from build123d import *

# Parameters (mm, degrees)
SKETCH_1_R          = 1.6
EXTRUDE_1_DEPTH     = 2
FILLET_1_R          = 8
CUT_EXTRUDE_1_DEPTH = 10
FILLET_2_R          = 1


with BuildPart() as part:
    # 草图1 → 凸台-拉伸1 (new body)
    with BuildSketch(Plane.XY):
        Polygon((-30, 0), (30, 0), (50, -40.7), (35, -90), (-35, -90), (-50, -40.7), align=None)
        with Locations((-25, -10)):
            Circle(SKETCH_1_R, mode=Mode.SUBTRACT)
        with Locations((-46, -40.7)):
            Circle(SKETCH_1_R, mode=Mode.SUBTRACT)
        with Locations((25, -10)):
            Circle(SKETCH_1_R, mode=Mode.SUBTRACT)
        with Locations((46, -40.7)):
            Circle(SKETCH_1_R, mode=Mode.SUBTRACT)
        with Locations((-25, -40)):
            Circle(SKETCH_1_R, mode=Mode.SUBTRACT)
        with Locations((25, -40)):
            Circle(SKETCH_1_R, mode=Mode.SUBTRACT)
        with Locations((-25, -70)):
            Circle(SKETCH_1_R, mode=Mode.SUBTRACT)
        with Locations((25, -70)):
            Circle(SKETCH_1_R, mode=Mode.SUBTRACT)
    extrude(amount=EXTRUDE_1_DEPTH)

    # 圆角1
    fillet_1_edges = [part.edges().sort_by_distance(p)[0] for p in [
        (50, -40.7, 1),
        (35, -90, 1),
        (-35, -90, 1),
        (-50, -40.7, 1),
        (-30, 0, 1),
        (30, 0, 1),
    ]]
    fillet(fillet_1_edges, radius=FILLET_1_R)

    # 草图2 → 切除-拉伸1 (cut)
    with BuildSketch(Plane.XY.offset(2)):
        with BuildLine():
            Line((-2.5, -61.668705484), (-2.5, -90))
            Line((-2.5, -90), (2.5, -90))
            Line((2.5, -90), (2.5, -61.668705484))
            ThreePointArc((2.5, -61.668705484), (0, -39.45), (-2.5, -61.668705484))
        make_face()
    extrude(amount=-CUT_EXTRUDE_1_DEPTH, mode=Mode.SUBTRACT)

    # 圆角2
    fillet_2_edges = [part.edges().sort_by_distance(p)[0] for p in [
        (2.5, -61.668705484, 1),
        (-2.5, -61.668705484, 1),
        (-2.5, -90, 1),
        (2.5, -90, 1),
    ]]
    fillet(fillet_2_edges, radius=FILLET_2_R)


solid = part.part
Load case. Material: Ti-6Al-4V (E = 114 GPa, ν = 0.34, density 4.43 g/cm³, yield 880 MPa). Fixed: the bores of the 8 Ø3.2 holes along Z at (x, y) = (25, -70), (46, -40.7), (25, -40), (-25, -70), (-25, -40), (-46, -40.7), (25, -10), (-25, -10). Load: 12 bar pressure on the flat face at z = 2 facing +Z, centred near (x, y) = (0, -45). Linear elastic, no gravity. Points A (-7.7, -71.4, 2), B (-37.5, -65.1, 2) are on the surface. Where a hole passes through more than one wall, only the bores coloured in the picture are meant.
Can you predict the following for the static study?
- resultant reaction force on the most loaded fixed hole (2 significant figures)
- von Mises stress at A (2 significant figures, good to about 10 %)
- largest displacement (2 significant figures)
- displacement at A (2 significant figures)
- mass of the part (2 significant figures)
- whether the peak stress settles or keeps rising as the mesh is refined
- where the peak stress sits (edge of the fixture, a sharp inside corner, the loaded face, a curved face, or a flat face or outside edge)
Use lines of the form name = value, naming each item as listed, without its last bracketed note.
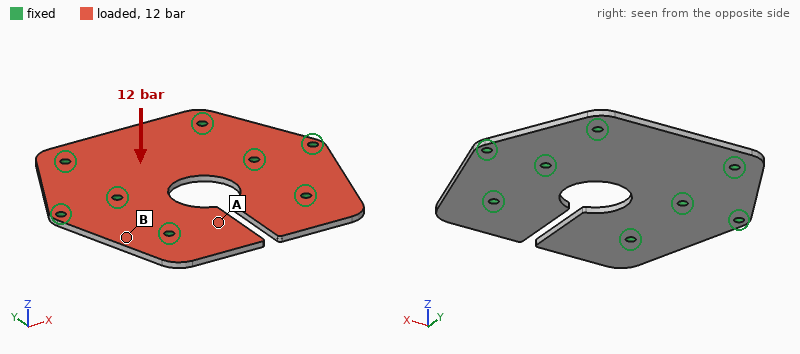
resultant reaction force on the most loaded fixed hole = 1.6 kN
von Mises stress at A = 99 MPa
largest displacement = 0.81 mm
displacement at A = 0.37 mm
mass of the part = 60 g
whether the peak stress settles or keeps rising as the mesh is refined = keeps rising
where the peak stress sits = edge of the fixture
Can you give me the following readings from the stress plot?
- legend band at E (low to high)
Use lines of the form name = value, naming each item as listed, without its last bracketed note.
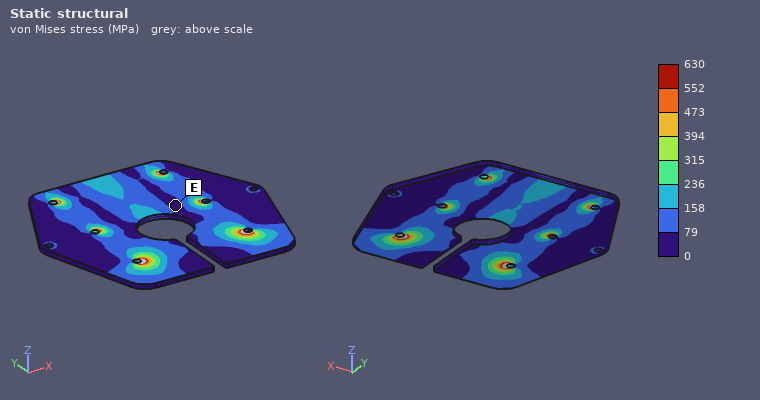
legend band at E = 0 to 79 MPa
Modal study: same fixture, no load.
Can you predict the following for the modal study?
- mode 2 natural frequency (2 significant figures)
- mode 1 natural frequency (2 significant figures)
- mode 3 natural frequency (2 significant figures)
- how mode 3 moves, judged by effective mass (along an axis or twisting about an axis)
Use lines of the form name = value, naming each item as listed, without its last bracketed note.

mode 2 natural frequency = 2800 Hz
mode 1 natural frequency = 2800 Hz
mode 3 natural frequency = 4000 Hz
how mode 3 moves, judged by effective mass = along Z
